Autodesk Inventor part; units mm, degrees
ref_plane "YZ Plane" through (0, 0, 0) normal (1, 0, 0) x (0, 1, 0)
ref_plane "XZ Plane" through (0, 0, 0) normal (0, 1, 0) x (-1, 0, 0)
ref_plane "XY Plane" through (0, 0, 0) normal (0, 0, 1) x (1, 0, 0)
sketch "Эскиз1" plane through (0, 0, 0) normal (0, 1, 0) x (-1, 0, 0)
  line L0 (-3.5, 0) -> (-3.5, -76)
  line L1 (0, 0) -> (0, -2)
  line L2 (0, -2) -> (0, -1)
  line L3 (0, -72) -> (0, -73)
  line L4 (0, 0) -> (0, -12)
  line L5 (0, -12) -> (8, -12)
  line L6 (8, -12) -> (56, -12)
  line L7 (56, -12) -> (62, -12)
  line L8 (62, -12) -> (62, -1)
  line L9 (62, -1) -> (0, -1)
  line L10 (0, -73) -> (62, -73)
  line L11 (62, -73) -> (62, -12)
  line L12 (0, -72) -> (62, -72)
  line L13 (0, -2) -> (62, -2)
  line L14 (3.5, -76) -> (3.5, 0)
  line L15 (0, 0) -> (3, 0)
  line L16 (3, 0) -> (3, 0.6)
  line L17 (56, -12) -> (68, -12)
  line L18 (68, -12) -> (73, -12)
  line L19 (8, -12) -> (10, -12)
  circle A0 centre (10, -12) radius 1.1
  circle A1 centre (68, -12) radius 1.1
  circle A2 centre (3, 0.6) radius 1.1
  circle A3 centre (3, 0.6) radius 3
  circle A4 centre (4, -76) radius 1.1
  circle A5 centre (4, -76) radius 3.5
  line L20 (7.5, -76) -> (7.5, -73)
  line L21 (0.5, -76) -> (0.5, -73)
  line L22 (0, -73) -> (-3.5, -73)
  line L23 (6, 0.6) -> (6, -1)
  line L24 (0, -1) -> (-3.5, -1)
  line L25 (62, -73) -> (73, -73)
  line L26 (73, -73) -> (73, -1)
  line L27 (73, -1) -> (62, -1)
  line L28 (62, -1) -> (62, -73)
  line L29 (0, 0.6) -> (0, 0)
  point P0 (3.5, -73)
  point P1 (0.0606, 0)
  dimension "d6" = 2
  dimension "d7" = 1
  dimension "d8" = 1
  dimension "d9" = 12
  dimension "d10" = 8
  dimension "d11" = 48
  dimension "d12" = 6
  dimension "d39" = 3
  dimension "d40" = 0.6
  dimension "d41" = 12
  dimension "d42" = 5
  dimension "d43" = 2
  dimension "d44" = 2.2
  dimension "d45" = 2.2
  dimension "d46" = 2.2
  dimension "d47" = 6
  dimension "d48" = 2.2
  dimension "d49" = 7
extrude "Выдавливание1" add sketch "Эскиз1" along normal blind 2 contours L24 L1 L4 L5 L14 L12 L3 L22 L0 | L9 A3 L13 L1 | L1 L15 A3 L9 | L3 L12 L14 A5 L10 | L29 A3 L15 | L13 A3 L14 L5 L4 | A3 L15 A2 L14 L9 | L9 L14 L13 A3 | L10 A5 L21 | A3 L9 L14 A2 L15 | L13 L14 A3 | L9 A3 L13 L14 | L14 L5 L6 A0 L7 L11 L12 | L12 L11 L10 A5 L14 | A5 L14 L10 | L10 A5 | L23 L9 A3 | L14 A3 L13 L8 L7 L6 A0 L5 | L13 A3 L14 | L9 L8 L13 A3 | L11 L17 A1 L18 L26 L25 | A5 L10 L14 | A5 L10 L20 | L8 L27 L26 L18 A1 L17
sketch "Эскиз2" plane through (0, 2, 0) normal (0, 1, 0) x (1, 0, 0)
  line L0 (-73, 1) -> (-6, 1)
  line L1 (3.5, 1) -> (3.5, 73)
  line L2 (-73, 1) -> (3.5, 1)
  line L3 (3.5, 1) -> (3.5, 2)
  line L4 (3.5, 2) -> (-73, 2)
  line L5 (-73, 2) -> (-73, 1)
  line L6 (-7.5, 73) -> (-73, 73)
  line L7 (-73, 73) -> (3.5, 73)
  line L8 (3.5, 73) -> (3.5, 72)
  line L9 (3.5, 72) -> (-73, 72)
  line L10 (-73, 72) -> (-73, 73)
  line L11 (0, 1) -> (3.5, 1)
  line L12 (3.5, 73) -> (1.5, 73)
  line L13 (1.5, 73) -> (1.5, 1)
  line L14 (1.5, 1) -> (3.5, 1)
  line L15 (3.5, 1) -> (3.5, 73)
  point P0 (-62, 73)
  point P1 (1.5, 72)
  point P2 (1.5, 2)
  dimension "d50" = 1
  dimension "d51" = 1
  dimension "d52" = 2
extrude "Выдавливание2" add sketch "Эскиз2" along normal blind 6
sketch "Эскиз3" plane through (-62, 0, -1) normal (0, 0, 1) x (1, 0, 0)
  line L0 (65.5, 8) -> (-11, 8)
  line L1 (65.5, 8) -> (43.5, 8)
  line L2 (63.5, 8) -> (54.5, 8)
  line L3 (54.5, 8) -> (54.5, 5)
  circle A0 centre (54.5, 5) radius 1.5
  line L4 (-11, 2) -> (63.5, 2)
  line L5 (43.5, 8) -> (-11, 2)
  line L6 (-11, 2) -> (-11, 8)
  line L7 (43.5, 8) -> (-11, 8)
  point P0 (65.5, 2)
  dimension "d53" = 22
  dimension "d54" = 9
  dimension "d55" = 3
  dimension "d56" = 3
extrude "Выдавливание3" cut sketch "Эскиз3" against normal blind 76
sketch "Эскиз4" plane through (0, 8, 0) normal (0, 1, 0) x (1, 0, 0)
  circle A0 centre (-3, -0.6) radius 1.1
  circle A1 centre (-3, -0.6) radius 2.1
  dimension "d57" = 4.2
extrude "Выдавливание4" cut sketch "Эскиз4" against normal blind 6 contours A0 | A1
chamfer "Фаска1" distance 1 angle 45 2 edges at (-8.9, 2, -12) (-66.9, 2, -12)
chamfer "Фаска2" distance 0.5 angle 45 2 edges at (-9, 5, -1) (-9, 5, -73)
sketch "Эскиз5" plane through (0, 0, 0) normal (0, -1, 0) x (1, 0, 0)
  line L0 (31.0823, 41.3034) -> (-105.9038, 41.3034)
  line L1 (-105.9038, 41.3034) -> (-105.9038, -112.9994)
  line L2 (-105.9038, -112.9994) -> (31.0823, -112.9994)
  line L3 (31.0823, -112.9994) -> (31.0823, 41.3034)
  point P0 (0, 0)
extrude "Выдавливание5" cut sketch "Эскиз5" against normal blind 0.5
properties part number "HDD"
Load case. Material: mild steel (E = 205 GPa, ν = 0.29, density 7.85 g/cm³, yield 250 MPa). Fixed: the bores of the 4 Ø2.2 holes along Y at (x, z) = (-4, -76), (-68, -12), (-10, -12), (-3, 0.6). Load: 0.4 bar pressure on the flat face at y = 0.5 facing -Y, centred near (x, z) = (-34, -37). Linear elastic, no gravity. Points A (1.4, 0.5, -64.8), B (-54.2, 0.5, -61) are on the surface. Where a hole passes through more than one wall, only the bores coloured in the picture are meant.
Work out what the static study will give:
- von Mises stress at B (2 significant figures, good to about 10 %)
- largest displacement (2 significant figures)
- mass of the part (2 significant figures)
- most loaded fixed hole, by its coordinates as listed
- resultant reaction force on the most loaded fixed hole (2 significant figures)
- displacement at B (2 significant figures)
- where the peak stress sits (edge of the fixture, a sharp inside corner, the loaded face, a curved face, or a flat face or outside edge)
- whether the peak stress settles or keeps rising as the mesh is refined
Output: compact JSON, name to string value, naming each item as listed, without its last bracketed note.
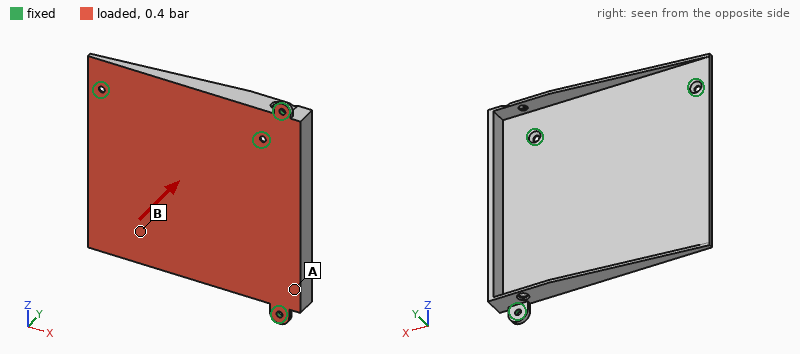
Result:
{"von Mises stress at B": "35 MPa", "largest displacement": "0.44 mm", "mass of the part": "76 g", "most loaded fixed hole, by its coordinates as listed": "(-10, -12)", "resultant reaction force on the most loaded fixed hole": "160 N", "displacement at B": "0.29 mm", "where the peak stress sits": "edge of the fixture", "whether the peak stress settles or keeps rising as the mesh is refined": "keeps rising"}
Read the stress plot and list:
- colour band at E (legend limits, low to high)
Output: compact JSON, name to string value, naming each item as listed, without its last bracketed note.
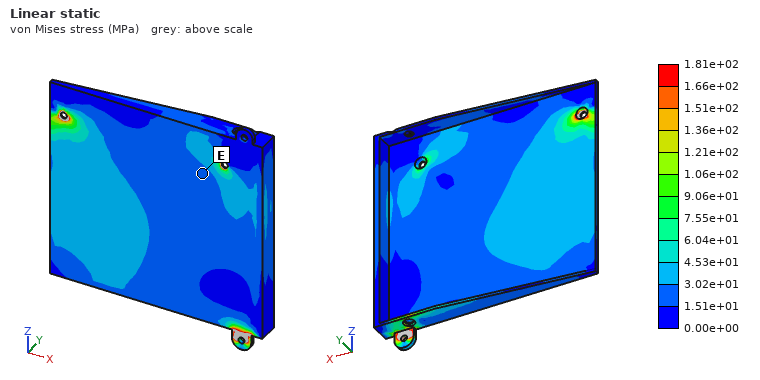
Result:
{"colour band at E": "1.51e+01 to 3.02e+01 MPa"}
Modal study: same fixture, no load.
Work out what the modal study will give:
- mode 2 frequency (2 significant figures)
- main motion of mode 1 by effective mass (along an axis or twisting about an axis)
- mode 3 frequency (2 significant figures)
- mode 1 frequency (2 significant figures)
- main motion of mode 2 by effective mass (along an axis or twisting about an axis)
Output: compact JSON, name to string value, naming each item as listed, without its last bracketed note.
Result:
{"mode 2 frequency": "1800 Hz", "main motion of mode 1 by effective mass": "along Y", "mode 3 frequency": "2200 Hz", "mode 1 frequency": "610 Hz", "main motion of mode 2 by effective mass": "along Y"}
